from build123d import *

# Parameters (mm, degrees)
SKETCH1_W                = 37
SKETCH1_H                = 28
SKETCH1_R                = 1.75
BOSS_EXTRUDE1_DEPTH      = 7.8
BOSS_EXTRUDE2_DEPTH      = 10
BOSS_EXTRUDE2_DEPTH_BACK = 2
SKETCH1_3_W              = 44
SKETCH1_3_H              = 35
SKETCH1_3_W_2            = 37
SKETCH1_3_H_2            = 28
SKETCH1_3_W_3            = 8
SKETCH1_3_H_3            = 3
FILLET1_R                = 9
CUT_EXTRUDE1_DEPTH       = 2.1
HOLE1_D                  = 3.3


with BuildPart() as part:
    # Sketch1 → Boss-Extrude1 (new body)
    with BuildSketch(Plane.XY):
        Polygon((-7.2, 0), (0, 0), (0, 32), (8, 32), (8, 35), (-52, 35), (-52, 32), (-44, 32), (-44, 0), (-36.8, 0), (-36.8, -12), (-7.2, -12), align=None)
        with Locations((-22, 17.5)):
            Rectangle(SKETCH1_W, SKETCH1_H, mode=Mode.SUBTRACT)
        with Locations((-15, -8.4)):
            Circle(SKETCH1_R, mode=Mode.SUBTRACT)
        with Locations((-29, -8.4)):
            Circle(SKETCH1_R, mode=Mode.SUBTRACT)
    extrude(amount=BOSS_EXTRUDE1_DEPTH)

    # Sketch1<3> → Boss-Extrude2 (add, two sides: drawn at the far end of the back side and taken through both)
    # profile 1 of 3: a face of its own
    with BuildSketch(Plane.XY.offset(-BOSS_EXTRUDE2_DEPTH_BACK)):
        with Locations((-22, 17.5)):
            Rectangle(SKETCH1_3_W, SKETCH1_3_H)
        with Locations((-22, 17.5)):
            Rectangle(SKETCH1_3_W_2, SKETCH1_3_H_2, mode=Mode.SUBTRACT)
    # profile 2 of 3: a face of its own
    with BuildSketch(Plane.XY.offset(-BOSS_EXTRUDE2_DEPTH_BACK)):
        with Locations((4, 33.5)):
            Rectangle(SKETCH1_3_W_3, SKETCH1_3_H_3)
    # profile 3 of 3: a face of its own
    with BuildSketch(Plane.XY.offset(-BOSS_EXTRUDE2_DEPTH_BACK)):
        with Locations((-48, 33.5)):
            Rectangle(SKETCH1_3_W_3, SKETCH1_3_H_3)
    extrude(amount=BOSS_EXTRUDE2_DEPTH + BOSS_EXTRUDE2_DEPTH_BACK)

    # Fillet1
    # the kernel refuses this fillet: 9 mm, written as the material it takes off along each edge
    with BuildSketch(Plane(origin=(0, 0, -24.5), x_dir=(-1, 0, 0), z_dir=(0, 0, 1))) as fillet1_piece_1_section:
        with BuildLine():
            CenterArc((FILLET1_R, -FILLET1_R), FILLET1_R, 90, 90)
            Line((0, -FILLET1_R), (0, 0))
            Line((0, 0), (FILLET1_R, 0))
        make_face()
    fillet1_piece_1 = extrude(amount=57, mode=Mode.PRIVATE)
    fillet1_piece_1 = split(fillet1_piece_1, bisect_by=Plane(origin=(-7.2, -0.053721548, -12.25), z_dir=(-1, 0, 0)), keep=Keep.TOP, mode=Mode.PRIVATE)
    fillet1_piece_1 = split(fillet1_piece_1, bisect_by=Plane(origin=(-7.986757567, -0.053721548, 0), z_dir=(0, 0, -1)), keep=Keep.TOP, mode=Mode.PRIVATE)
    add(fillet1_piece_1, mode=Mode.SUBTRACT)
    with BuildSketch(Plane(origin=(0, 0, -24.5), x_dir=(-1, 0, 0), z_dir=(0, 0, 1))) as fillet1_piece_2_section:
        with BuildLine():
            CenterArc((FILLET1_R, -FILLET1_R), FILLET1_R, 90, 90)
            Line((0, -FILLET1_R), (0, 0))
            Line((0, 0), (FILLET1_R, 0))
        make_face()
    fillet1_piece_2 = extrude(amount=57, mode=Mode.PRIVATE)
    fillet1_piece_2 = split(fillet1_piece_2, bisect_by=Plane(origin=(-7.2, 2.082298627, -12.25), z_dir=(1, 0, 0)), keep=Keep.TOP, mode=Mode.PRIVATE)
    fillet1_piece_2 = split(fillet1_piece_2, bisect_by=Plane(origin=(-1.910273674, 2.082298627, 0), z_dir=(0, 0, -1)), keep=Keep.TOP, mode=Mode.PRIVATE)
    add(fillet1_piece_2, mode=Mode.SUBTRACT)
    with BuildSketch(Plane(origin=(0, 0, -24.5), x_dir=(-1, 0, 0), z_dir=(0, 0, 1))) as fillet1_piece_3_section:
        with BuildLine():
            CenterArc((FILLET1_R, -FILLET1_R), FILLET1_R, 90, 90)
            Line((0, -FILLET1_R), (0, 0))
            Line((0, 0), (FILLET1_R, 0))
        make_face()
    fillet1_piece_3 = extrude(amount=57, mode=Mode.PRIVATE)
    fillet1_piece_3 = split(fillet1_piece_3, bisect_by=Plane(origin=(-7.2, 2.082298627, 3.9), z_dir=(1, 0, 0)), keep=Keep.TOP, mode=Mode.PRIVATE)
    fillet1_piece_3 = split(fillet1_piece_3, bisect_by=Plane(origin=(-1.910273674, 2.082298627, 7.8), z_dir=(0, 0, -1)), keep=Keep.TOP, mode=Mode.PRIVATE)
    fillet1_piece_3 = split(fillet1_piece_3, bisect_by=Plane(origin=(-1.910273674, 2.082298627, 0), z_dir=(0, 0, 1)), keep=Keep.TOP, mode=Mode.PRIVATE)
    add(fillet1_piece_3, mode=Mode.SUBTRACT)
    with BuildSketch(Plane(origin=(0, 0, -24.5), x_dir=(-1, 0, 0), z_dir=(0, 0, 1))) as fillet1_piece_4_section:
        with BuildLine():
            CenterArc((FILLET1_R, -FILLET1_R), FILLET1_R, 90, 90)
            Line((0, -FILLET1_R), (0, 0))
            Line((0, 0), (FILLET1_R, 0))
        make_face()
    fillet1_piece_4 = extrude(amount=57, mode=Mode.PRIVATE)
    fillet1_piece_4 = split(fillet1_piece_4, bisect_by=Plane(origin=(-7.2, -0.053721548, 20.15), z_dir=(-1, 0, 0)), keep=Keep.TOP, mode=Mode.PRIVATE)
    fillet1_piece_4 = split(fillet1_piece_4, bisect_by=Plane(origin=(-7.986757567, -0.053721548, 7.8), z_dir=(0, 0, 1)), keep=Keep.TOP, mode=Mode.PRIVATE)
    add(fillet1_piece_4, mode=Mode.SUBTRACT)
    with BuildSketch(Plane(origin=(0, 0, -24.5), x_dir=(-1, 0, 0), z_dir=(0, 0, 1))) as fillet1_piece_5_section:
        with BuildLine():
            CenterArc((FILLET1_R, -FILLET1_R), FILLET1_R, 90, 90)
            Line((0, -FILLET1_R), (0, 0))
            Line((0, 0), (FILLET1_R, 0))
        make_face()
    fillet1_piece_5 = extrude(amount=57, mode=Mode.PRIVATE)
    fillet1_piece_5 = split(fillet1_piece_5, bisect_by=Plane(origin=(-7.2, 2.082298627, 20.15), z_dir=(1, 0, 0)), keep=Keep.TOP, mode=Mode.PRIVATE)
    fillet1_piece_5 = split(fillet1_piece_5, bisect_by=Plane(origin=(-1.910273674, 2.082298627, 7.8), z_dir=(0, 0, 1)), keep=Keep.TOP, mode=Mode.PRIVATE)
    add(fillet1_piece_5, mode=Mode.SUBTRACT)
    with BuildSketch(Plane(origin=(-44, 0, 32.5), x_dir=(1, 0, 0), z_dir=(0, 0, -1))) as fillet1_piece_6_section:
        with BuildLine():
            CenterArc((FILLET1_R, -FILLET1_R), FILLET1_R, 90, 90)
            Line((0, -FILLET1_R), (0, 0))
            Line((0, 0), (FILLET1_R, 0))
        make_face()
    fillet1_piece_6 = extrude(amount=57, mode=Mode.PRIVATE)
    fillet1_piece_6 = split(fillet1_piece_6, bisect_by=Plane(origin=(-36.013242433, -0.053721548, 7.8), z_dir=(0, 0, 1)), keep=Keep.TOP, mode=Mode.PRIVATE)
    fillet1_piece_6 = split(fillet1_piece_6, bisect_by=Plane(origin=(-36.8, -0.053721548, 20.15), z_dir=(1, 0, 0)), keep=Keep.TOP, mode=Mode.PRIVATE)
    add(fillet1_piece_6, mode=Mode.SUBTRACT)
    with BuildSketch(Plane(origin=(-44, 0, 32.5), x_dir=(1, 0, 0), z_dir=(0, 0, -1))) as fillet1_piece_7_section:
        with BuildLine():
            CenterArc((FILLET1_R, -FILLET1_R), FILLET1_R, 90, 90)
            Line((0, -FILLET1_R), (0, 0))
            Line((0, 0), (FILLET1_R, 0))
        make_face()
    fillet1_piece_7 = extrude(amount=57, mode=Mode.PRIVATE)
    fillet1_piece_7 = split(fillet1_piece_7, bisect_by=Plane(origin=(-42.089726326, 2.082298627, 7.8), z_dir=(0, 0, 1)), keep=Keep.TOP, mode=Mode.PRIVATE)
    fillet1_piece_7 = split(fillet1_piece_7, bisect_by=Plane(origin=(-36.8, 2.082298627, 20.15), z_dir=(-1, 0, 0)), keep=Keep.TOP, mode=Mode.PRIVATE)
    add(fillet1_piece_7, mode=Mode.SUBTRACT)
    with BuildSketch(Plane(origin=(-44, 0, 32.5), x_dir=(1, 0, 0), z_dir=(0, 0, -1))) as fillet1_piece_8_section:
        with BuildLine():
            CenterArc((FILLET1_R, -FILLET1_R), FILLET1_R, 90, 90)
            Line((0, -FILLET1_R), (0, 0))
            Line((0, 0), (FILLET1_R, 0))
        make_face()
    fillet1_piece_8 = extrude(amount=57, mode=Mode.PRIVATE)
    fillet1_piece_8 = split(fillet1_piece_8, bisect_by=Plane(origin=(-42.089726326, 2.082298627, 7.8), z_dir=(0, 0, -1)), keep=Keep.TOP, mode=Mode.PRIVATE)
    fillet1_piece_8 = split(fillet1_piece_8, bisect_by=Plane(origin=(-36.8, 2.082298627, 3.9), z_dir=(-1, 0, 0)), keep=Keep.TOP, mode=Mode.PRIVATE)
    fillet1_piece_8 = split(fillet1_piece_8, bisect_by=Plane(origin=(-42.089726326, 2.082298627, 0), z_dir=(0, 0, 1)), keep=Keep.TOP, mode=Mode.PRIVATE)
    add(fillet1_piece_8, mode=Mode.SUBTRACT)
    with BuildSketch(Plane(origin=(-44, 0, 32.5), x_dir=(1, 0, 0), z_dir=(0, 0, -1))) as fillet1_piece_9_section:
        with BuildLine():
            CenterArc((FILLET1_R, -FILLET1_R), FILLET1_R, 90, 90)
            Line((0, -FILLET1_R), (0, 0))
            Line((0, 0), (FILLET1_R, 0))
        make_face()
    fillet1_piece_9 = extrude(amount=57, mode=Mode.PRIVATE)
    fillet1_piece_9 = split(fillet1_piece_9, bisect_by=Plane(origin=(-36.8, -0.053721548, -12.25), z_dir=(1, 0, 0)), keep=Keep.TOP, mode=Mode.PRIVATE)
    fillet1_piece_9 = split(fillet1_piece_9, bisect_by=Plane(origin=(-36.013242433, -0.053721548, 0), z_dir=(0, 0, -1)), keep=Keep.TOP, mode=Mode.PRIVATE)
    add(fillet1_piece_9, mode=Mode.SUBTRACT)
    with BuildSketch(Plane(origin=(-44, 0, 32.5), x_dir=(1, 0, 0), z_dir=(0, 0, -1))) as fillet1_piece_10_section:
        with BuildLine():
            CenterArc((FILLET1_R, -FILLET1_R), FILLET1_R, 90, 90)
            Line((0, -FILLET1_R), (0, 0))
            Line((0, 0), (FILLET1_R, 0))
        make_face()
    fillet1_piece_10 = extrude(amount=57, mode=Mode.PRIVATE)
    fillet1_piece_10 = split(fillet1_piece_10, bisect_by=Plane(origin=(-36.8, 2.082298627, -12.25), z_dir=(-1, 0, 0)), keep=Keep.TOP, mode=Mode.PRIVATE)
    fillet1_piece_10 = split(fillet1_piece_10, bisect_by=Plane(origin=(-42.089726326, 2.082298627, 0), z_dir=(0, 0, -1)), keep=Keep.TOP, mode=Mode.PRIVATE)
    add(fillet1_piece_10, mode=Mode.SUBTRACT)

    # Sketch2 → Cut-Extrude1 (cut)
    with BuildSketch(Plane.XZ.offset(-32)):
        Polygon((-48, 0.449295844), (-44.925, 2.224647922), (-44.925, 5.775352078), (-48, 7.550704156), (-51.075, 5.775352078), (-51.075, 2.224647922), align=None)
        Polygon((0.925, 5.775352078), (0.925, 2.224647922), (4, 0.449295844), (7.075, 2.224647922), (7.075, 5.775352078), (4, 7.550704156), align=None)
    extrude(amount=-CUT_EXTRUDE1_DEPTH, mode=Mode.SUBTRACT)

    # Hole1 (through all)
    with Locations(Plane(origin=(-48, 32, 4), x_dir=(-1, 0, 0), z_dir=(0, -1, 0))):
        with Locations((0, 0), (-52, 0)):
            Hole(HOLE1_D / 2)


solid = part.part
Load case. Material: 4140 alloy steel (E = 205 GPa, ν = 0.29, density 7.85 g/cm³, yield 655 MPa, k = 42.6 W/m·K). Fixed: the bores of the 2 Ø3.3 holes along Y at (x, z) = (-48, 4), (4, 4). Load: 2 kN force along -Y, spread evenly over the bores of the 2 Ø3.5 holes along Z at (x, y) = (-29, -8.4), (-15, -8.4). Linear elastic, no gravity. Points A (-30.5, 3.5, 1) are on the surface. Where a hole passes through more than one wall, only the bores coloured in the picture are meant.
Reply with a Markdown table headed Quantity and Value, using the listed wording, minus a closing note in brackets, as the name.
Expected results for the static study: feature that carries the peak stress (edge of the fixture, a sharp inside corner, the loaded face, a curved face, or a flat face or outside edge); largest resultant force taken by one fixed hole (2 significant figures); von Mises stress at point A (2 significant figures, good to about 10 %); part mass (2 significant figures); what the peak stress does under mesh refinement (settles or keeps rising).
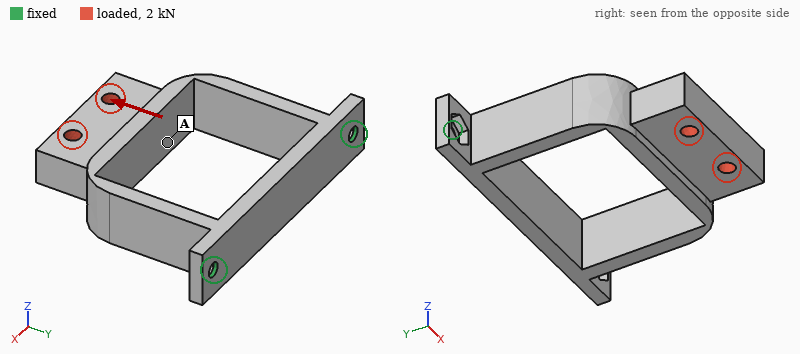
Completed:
| Quantity | Value |
|---|---|
| feature that carries the peak stress | edge of the fixture |
| largest resultant force taken by one fixed hole | 1.2 kN |
| von Mises stress at point A | 49 MPa |
| part mass | 68 g |
| what the peak stress does under mesh refinement | keeps rising |
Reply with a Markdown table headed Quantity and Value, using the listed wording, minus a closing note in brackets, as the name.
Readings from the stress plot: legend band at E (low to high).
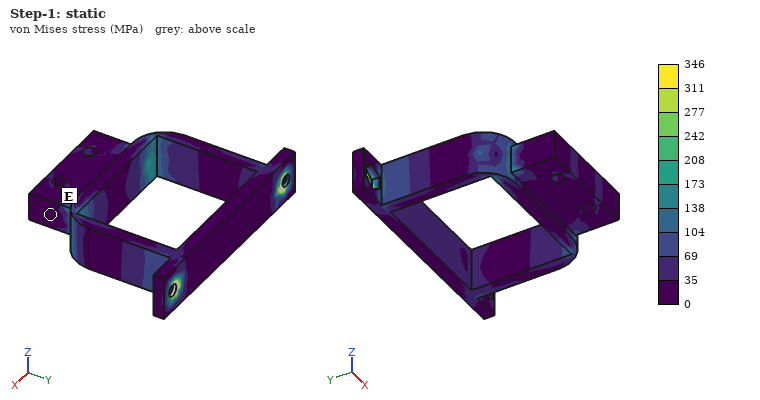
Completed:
| Quantity | Value |
|---|---|
| legend band at E | 0 to 35 MPa |
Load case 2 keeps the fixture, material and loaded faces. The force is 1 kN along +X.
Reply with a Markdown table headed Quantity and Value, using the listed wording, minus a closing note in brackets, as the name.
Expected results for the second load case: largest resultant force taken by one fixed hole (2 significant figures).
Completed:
| Quantity | Value |
|---|---|
| largest resultant force taken by one fixed hole | 960 N |
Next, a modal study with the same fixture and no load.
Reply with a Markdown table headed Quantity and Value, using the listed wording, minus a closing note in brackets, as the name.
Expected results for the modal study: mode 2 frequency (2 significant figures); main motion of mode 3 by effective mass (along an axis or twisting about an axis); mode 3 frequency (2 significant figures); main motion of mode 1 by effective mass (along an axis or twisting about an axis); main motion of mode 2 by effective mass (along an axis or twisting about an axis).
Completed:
| Quantity | Value |
|---|---|
| mode 2 frequency | 1300 Hz |
| main motion of mode 3 by effective mass | twisting about Y |
| mode 3 frequency | 3500 Hz |
| main motion of mode 1 by effective mass | along Z |
| main motion of mode 2 by effective mass | along X |
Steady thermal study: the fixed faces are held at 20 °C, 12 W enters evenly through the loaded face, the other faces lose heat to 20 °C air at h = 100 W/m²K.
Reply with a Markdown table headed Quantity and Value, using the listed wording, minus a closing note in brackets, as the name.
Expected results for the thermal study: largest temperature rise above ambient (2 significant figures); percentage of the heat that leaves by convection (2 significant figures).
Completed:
| Quantity | Value |
|---|---|
| largest temperature rise above ambient | 50 K |
| percentage of the heat that leaves by convection | 91 % |
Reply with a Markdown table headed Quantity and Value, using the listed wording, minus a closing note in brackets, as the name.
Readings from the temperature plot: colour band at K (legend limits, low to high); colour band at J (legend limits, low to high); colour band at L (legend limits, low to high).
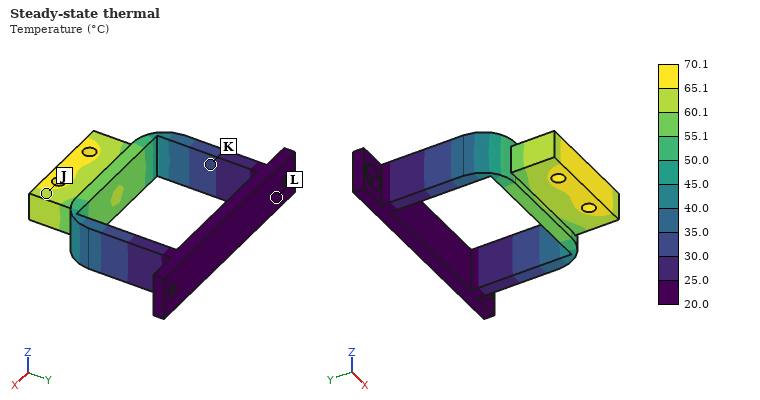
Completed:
| Quantity | Value |
|---|---|
| colour band at K | 30.0 to 35.0 °C |
| colour band at J | 60.1 to 65.1 °C |
| colour band at L | 20.0 to 25.0 °C |
